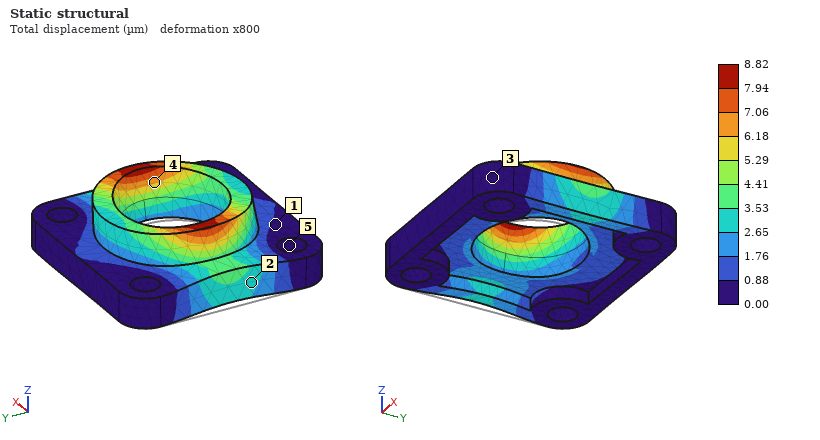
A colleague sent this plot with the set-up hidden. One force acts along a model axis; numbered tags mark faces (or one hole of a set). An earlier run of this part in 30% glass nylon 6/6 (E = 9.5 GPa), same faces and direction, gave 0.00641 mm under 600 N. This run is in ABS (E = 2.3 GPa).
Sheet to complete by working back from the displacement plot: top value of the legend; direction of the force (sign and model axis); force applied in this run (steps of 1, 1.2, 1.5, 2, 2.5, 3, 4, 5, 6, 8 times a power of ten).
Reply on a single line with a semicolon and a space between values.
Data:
8.82 µm; +X; 200 N
